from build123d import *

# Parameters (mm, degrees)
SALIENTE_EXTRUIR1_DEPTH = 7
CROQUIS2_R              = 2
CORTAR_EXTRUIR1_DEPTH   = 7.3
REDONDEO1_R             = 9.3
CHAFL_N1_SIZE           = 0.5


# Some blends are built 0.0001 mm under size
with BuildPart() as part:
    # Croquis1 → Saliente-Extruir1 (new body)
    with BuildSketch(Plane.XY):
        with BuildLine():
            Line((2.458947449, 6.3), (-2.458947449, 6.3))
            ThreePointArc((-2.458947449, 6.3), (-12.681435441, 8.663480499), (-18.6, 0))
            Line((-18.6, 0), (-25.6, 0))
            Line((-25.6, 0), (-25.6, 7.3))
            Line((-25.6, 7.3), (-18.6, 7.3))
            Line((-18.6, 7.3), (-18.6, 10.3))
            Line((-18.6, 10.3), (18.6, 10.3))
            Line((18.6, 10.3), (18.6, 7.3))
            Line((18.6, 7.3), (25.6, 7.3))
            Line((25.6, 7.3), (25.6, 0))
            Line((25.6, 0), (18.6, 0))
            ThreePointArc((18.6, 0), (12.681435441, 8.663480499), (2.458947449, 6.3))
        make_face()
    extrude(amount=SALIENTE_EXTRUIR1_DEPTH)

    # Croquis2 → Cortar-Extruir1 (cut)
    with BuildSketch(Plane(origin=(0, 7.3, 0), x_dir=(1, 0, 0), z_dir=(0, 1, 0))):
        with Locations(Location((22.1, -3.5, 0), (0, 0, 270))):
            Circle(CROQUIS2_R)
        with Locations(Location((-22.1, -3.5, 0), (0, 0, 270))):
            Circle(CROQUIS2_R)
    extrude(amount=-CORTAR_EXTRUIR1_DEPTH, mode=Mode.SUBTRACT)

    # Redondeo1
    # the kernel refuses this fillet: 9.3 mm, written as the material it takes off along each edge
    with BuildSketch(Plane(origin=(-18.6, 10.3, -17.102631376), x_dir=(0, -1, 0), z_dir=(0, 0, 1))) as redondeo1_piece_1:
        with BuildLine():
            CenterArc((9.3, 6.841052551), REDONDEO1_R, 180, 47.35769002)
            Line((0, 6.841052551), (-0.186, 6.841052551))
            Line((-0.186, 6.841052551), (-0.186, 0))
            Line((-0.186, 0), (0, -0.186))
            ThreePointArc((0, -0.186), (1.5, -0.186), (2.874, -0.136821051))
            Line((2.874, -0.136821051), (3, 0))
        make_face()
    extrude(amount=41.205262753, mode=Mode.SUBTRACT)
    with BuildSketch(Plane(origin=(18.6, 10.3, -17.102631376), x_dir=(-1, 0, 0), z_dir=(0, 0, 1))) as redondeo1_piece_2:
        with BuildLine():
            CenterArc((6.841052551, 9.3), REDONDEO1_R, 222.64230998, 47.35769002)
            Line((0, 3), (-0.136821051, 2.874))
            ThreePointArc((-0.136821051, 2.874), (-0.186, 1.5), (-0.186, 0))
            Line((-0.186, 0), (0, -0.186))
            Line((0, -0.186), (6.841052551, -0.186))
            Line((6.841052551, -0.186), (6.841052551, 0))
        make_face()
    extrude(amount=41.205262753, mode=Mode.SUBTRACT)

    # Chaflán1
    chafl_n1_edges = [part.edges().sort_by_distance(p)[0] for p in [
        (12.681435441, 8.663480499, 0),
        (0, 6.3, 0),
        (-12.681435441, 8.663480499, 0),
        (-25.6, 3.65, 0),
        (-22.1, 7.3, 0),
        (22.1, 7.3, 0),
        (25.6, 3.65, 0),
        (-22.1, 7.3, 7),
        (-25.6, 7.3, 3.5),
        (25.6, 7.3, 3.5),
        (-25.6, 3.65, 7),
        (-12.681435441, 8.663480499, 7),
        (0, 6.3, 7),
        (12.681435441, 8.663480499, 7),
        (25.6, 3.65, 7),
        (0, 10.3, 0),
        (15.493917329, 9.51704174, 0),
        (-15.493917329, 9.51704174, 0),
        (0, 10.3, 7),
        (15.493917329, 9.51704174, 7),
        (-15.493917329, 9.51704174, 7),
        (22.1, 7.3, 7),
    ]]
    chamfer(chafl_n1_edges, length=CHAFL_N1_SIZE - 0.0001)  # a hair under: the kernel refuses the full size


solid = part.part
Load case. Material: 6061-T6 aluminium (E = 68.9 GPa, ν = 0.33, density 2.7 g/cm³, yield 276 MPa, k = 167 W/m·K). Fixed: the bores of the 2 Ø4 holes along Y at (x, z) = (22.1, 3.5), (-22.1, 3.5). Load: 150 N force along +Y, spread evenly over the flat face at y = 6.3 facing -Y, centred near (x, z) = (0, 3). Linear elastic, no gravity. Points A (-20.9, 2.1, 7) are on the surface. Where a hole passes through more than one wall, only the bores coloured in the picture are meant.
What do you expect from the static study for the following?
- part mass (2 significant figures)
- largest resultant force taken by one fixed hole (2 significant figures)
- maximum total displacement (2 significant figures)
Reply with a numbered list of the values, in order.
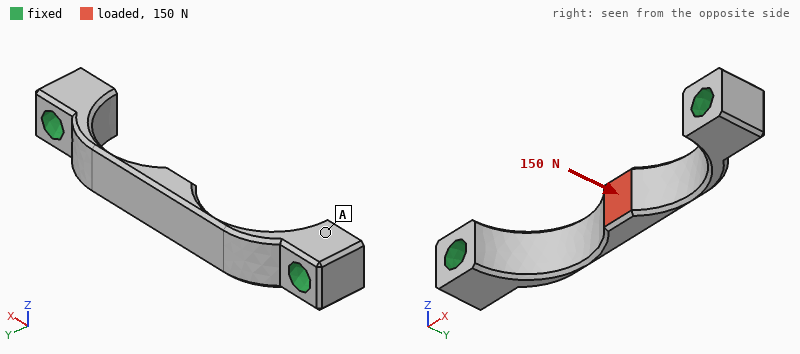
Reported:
1. 3.0 g
2. 160 N
3. 77 µm
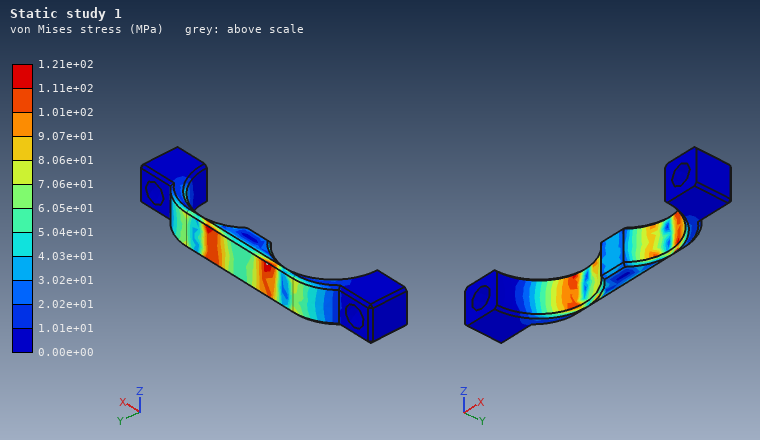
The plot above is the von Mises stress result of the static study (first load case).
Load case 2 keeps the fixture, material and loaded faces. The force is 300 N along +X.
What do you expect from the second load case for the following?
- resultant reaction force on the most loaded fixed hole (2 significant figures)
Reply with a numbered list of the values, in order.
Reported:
1. 160 N
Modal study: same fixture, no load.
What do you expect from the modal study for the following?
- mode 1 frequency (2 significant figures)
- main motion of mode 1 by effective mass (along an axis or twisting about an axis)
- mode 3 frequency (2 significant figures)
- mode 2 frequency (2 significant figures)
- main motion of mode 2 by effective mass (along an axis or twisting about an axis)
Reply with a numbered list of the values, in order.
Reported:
1. 8000 Hz
2. along Y
3. 14 kHz
4. 10 kHz
5. along Z
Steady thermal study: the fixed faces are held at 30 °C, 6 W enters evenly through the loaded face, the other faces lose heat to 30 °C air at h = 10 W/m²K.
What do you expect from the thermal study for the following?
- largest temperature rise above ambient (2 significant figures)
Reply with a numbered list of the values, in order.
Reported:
1. 32 K
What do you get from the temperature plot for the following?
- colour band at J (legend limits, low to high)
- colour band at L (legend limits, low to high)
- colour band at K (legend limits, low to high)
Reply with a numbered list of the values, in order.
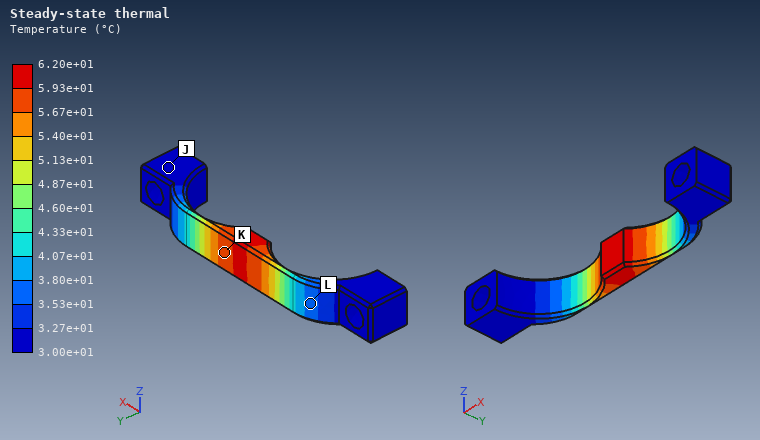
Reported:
1. 3.00e+01 to 3.27e+01 °C
2. 3.53e+01 to 3.80e+01 °C
3. 5.67e+01 to 5.93e+01 °C
